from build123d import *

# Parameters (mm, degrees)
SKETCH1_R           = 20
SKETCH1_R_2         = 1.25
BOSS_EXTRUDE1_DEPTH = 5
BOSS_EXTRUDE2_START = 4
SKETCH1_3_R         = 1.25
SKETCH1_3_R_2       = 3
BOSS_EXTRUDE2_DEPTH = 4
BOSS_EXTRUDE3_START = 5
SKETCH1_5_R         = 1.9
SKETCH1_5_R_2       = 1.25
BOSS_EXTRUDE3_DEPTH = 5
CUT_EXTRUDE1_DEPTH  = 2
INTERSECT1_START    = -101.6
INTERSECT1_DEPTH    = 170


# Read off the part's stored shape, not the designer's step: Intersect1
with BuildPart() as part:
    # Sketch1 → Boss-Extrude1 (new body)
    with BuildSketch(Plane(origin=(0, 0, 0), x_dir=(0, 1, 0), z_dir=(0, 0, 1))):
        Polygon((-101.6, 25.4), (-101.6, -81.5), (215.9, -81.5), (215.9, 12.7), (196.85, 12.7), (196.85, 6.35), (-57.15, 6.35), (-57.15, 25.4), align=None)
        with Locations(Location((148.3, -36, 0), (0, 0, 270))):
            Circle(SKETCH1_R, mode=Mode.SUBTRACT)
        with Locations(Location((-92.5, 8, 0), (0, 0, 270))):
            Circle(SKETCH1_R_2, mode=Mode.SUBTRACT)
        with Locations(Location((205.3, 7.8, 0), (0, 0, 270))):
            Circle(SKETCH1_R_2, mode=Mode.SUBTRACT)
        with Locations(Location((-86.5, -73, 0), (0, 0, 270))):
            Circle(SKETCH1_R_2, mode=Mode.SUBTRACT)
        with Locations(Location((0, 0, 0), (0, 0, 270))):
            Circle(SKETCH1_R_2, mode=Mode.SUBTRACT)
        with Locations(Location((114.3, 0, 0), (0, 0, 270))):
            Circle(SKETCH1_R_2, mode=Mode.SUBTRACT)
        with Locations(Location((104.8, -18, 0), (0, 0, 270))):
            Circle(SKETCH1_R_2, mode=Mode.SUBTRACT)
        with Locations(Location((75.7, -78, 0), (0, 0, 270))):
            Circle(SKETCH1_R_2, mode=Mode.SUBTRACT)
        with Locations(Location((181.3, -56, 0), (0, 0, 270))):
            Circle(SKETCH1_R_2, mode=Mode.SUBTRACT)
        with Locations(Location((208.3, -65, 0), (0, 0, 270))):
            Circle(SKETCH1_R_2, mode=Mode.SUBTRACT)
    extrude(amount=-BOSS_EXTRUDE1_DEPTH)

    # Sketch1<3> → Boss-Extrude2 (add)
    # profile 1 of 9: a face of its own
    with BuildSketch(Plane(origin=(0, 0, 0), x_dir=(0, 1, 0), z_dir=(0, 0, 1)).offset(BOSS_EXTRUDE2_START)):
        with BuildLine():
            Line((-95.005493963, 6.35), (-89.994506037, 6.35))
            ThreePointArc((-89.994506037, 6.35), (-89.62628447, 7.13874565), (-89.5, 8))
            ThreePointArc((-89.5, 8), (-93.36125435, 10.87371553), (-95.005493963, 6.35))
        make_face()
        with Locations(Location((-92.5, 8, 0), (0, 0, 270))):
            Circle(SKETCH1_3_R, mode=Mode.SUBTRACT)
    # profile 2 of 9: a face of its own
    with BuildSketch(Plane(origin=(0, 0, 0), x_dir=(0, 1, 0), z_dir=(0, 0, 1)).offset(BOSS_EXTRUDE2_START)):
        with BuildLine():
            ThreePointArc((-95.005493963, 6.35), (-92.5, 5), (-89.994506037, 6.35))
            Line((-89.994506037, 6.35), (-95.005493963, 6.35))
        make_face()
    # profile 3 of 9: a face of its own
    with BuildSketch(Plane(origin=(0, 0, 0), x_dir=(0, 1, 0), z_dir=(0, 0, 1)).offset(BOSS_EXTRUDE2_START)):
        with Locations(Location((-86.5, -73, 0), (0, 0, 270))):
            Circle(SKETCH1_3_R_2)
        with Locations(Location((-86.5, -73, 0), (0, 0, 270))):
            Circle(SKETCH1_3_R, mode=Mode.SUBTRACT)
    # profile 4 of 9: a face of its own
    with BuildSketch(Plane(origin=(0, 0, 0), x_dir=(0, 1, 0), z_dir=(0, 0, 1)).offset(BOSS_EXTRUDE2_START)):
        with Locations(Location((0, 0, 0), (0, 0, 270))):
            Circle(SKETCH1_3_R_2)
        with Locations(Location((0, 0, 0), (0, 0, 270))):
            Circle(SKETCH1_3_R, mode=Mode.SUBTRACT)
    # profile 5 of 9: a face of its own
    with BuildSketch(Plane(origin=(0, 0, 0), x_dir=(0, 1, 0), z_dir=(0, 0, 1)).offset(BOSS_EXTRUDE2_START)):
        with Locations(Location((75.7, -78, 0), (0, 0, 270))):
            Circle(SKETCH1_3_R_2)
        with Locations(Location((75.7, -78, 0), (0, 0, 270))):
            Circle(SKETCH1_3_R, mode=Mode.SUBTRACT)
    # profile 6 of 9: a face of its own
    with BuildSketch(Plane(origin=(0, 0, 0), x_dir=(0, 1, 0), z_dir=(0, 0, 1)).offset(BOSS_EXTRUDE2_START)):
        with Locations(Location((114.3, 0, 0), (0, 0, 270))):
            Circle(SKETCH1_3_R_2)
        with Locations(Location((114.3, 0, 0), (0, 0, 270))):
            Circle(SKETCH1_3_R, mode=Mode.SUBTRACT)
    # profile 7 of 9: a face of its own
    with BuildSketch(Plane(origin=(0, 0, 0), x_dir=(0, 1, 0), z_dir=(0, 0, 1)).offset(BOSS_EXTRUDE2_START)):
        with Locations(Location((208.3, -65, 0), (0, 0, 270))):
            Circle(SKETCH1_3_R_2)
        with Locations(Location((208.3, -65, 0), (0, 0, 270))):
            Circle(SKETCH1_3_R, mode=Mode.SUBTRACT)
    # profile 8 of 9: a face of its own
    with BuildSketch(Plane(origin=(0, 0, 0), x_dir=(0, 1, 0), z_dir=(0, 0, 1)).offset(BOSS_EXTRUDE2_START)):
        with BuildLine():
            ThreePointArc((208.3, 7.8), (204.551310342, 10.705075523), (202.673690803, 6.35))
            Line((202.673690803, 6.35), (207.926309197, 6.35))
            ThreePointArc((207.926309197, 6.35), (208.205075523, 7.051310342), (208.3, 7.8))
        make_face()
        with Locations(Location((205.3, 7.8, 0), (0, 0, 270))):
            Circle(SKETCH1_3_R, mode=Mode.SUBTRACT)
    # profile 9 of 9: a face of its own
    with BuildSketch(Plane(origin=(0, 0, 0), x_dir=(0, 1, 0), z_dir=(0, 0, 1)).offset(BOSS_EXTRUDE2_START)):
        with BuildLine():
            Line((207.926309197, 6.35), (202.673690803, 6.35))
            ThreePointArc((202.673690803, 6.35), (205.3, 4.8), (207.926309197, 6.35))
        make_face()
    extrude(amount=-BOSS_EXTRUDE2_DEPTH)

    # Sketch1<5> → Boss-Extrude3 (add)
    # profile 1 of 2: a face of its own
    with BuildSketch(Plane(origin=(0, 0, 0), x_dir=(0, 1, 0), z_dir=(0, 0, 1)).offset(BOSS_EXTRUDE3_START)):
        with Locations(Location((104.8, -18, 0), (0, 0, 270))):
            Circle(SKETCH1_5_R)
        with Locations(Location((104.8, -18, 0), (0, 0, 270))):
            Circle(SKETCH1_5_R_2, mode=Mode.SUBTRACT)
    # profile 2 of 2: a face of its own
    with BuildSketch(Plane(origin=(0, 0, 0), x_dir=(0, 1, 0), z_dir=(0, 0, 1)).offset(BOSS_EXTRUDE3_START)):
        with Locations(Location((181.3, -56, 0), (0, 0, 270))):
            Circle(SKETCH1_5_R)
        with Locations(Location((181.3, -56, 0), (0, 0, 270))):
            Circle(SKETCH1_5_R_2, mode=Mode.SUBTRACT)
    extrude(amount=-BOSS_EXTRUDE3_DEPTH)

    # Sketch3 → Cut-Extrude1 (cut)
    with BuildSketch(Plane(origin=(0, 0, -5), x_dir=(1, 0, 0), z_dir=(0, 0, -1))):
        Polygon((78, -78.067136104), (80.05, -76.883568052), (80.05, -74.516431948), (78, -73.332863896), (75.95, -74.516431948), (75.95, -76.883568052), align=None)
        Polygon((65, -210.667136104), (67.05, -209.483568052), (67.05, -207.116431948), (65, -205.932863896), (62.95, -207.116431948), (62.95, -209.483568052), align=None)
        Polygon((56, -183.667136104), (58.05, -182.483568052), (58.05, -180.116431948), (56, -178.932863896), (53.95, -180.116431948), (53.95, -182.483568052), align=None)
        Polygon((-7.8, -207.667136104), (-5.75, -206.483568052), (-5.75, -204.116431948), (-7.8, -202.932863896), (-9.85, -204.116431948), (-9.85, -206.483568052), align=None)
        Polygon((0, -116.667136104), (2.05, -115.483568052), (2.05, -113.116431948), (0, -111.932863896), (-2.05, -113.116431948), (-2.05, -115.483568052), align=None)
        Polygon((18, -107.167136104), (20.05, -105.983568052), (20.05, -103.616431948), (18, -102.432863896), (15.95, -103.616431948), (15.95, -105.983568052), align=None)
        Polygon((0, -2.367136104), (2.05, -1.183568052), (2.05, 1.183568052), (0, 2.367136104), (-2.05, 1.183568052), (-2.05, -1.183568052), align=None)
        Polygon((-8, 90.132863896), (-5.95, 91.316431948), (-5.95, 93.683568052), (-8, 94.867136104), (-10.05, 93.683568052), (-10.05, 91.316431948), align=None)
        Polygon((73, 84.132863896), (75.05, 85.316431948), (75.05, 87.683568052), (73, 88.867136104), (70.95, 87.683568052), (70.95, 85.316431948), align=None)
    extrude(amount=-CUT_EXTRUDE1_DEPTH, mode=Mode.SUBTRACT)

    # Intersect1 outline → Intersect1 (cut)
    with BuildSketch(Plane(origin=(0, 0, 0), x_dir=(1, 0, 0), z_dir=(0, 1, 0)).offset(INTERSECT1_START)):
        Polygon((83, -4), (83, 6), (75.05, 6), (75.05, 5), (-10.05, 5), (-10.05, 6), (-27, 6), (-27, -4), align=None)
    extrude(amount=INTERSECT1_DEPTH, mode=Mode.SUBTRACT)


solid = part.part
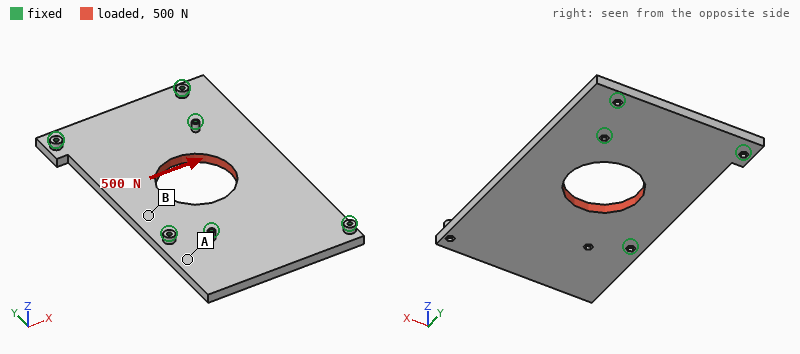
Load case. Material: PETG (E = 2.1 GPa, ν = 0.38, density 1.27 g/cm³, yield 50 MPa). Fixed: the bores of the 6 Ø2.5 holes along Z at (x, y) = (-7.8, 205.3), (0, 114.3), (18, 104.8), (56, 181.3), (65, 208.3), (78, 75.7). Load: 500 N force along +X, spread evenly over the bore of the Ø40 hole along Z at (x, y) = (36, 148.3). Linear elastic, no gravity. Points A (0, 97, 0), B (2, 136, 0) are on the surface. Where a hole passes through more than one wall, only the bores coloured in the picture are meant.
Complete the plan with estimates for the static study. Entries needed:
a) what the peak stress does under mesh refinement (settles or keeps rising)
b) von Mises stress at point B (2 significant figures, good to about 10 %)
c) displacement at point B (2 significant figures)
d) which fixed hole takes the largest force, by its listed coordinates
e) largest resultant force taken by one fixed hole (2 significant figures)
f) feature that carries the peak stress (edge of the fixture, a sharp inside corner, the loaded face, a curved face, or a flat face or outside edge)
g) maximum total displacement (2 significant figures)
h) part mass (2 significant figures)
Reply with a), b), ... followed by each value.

a) keeps rising
b) 0.86 MPa
c) 35 µm
d) (56, 181.3)
e) 170 N
f) edge of the fixture
g) 46 µm
h) 75 g
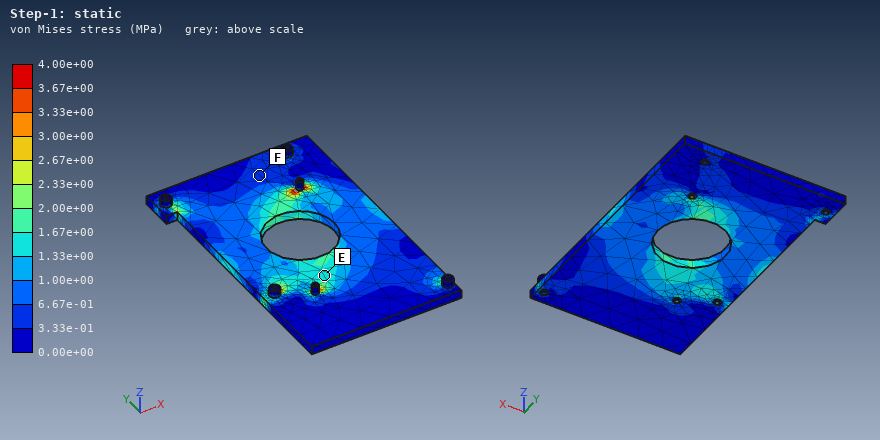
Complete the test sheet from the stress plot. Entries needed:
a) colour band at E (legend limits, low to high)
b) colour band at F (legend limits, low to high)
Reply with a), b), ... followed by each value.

a) 1.33e+00 to 1.67e+00 MPa
b) 3.33e-01 to 6.67e-01 MPa
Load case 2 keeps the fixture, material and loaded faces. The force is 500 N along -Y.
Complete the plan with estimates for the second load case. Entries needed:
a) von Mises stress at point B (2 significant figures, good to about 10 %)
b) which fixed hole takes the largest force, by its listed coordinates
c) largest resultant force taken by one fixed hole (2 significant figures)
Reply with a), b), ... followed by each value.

a) 0.80 MPa
b) (56, 181.3)
c) 130 N
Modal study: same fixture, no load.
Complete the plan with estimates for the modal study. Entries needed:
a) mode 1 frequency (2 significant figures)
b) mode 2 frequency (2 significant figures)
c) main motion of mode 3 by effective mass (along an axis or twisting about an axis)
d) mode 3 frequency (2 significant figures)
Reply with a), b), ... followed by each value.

a) 510 Hz
b) 670 Hz
c) along Z
d) 770 Hz
